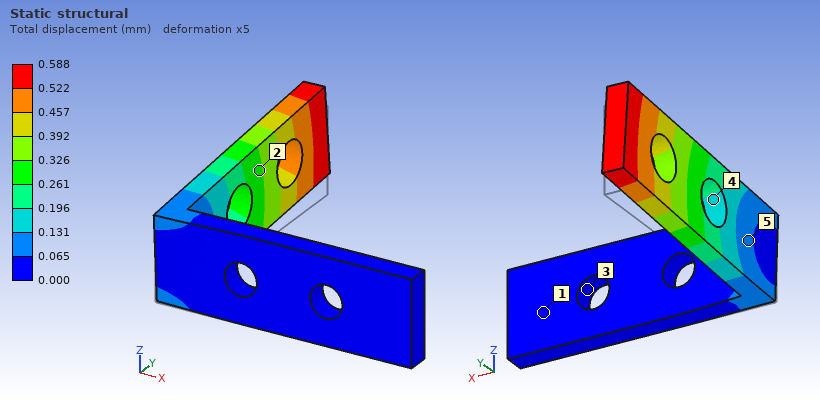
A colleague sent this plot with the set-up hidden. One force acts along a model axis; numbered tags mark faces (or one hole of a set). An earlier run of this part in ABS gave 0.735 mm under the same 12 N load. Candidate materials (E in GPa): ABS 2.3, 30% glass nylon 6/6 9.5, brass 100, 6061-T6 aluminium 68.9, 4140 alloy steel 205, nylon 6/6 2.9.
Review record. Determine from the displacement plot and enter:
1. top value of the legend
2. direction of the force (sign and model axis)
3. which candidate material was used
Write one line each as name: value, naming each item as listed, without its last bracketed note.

top value of the legend: 0.588 mm
direction of the force: +Z
which candidate material was used: nylon 6/6
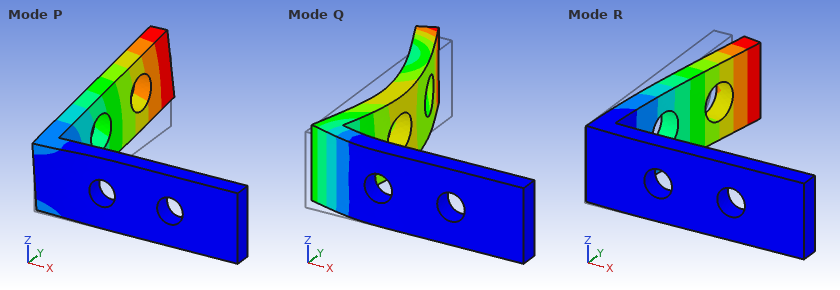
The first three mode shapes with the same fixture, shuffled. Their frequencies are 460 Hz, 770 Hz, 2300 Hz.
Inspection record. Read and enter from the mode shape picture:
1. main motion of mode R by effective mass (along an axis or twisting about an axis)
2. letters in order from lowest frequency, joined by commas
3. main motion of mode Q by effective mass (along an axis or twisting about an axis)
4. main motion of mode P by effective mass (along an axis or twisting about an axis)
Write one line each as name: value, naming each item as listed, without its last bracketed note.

main motion of mode R by effective mass: along X
letters in order from lowest frequency, joined by commas: R, P, Q
main motion of mode Q by effective mass: along Y
main motion of mode P by effective mass: along Z
